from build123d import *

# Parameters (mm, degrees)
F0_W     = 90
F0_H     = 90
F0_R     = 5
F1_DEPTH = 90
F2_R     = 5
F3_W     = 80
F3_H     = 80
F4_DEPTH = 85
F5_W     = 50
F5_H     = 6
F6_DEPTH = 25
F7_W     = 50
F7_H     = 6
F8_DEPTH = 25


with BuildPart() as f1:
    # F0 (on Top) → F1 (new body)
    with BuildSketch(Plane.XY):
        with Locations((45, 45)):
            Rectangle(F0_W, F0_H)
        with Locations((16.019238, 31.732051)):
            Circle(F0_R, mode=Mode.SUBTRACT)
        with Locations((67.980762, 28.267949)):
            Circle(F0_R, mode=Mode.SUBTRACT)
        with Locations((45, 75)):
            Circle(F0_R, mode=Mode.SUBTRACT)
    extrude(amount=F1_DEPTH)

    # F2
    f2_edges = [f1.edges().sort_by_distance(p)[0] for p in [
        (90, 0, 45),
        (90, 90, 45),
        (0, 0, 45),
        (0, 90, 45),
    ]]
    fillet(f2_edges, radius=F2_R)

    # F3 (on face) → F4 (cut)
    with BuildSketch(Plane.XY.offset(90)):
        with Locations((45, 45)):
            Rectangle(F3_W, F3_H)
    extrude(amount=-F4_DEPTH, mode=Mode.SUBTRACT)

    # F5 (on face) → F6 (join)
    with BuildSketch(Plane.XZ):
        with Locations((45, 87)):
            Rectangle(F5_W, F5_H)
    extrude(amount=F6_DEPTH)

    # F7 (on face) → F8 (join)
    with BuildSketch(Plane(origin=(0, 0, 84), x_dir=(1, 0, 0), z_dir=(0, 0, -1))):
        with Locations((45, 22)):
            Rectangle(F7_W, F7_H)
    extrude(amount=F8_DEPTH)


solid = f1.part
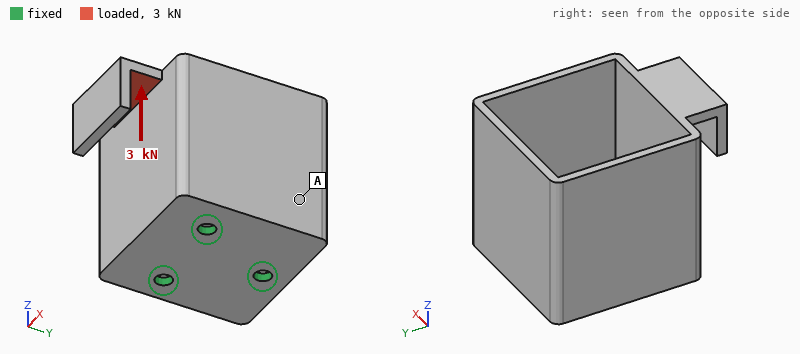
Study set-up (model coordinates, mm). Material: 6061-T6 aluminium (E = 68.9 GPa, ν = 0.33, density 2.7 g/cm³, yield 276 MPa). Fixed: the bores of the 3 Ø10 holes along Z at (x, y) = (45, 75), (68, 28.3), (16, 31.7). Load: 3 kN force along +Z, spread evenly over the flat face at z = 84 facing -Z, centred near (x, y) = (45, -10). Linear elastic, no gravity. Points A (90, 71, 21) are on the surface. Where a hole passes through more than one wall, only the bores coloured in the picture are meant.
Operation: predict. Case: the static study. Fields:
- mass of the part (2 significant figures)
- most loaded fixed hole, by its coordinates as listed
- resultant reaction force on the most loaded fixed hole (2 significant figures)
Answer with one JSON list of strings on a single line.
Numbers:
["530 g", "(68, 28.3)", "2.5 kN"]
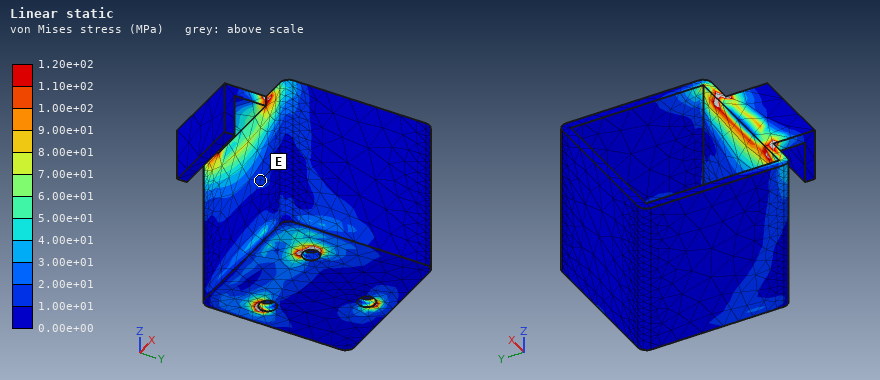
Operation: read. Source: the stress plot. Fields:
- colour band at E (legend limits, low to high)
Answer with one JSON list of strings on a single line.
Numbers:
["1.00e+01 to 2.00e+01 MPa"]
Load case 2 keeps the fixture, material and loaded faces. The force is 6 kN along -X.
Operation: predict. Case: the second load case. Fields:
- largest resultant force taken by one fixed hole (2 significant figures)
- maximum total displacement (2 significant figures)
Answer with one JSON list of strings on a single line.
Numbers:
["8.6 kN", "0.56 mm"]
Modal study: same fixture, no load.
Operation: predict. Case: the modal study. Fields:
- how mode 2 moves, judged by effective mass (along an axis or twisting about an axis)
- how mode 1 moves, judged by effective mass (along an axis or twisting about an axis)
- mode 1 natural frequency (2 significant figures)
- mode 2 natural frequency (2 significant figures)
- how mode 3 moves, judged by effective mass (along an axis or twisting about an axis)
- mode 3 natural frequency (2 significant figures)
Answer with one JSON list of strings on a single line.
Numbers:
["along Y", "along X", "1100 Hz", "1300 Hz", "along X", "1400 Hz"]
